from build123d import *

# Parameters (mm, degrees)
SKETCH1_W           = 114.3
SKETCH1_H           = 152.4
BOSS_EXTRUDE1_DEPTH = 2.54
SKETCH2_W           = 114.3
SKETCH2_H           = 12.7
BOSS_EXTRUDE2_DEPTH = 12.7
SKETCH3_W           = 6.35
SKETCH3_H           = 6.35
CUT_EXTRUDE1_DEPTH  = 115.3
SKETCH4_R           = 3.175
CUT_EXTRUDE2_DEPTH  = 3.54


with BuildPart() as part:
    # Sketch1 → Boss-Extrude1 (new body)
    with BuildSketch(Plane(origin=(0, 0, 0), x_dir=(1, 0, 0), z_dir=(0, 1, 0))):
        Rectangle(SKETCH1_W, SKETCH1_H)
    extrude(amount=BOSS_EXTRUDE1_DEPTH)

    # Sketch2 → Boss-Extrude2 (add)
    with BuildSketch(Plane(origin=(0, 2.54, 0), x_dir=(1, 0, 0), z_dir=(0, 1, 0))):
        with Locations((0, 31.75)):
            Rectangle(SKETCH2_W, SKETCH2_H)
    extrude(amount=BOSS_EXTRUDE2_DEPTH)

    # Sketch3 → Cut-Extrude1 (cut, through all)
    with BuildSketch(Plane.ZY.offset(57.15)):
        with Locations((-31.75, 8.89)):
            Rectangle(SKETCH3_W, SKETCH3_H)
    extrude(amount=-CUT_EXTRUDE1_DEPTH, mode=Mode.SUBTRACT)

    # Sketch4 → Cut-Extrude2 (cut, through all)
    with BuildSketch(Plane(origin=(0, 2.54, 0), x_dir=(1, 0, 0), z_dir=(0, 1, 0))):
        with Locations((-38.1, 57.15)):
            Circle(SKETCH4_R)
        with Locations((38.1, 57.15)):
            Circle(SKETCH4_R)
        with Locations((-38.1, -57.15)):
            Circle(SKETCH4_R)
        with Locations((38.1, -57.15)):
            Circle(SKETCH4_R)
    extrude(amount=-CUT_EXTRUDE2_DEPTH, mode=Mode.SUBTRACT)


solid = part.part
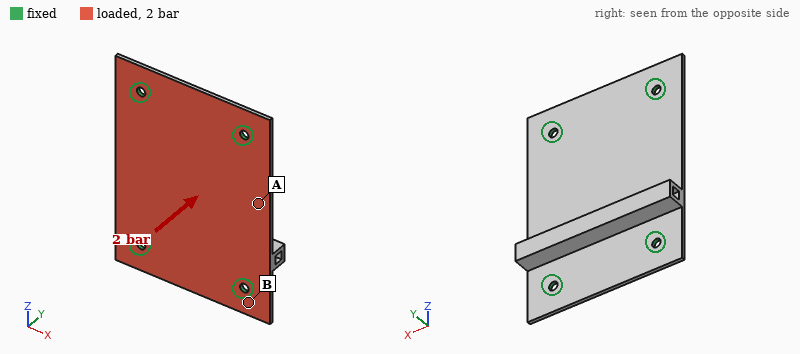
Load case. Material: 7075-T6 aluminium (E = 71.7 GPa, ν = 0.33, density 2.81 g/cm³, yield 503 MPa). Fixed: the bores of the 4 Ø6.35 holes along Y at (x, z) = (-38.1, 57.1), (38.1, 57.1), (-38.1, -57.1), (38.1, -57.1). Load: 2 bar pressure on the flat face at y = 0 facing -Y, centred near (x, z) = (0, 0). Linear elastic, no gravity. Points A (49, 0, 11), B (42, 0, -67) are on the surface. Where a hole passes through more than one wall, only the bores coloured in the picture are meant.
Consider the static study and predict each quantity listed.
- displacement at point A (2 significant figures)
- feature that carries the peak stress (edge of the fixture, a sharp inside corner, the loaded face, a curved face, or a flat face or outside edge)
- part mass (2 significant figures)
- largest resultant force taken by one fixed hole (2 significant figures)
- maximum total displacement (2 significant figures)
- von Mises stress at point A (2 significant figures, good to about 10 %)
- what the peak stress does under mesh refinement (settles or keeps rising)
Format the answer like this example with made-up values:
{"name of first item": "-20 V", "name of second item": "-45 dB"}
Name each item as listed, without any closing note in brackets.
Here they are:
{"displacement at point A": "0.90 mm", "feature that carries the peak stress": "edge of the fixture", "part mass": "160 g", "largest resultant force taken by one fixed hole": "880 N", "maximum total displacement": "1.0 mm", "von Mises stress at point A": "95 MPa", "what the peak stress does under mesh refinement": "keeps rising"}
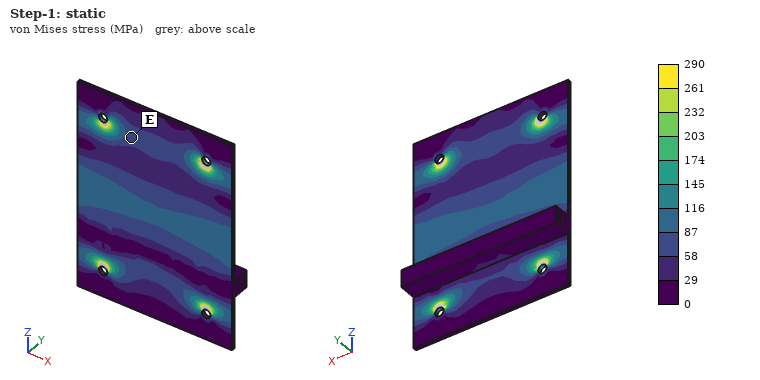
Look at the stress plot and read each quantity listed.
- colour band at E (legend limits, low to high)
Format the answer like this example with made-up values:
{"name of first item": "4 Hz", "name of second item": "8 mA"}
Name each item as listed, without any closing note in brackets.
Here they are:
{"colour band at E": "58 to 87 MPa"}
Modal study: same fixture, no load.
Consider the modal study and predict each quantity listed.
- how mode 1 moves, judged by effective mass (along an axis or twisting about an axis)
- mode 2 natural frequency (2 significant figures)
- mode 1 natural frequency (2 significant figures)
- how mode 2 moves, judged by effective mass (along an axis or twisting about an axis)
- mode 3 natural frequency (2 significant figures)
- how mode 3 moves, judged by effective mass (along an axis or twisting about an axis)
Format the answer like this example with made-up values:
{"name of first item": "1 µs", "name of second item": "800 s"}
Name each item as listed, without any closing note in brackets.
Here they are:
{"how mode 1 moves, judged by effective mass": "along Y", "mode 2 natural frequency": "1600 Hz", "mode 1 natural frequency": "830 Hz", "how mode 2 moves, judged by effective mass": "twisting about Z", "mode 3 natural frequency": "2100 Hz", "how mode 3 moves, judged by effective mass": "twisting about X"}
